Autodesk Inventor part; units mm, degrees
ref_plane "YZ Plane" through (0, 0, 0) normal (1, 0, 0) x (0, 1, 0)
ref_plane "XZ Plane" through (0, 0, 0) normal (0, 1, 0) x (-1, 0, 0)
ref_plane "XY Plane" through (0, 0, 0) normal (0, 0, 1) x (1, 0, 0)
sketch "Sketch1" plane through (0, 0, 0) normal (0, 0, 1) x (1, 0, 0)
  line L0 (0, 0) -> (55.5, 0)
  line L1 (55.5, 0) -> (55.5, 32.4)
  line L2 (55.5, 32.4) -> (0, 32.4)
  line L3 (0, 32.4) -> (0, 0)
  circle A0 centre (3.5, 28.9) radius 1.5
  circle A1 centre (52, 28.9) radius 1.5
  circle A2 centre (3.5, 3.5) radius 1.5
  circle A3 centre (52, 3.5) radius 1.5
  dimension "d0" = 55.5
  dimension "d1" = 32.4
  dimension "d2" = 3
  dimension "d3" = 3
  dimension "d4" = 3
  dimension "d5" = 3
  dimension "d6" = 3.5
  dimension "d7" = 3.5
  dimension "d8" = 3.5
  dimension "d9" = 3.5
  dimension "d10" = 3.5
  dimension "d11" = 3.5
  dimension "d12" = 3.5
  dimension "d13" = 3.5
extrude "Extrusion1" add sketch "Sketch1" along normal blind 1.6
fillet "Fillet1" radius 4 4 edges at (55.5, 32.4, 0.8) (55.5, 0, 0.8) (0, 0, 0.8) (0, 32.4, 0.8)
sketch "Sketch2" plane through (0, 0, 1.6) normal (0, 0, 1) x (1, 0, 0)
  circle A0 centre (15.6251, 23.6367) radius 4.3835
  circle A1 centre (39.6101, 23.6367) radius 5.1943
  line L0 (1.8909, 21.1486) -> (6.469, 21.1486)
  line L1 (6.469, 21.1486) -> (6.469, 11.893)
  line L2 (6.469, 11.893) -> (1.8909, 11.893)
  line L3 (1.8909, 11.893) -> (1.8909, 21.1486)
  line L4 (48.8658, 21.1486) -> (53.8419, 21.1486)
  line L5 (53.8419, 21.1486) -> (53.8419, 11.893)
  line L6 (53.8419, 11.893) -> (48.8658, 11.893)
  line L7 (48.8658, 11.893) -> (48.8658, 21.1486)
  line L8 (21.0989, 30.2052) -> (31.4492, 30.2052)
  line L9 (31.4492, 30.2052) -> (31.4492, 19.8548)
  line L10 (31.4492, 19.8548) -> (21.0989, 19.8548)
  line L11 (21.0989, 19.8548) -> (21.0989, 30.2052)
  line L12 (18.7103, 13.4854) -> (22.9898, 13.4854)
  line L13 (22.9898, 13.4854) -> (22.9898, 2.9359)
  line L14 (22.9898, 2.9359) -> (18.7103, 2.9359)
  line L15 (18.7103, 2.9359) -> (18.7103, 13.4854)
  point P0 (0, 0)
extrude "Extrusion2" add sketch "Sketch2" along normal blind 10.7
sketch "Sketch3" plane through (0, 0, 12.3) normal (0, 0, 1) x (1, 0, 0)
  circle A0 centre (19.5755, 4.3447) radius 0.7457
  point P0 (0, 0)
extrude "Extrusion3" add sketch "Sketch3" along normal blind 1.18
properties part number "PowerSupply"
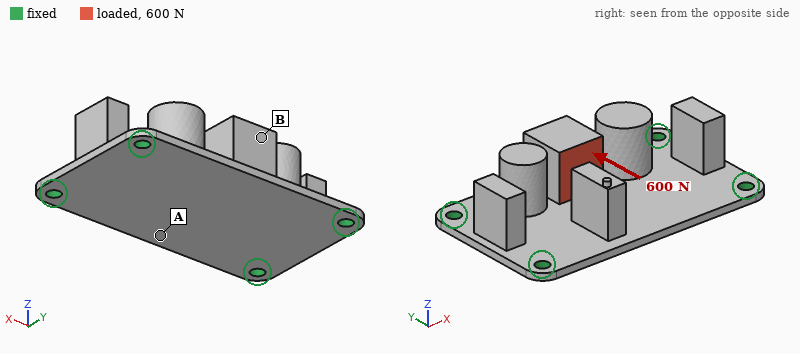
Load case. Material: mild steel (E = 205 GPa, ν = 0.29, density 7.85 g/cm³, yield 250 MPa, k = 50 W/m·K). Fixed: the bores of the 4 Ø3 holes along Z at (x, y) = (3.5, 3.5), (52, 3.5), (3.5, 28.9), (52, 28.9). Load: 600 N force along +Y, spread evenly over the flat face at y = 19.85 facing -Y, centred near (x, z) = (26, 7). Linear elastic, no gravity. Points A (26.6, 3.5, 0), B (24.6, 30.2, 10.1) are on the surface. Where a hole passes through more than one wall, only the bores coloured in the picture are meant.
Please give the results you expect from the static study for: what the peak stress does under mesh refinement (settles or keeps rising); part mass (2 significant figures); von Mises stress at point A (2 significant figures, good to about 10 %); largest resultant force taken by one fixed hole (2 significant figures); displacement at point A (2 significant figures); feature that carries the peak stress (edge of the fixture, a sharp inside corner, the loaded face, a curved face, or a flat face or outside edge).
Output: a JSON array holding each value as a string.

["keeps rising", "54 g", "36 MPa", "240 N", "29 µm", "edge of the fixture"]
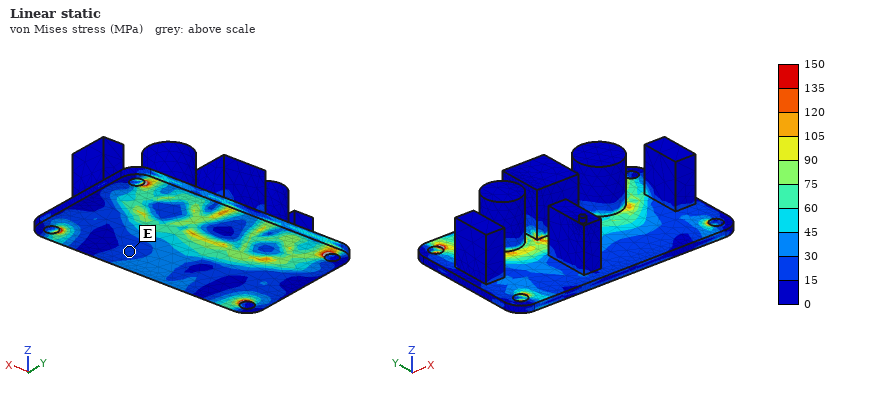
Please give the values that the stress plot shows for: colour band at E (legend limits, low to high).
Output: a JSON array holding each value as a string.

["15 to 30 MPa"]
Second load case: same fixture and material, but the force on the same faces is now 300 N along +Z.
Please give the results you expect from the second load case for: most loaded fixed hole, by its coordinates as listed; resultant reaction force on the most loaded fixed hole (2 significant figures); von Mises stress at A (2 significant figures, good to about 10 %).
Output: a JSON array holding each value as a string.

["(3.5, 28.9)", "130 N", "53 MPa"]
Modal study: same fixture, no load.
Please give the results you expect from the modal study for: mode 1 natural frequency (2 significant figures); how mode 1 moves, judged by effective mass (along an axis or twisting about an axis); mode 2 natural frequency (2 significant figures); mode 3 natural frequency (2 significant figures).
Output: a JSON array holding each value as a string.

["2200 Hz", "along Z", "3500 Hz", "5200 Hz"]
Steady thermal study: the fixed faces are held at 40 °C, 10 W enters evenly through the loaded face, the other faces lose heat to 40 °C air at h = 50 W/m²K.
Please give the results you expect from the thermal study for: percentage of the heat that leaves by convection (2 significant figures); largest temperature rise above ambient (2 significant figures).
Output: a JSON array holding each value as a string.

["45 %", "52 K"]
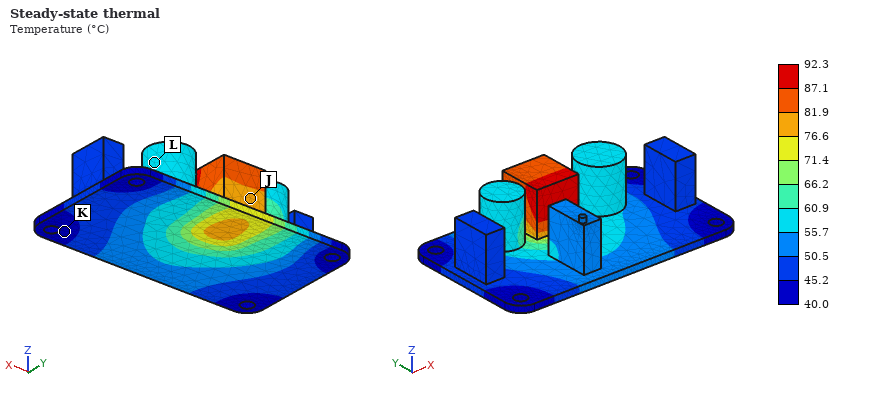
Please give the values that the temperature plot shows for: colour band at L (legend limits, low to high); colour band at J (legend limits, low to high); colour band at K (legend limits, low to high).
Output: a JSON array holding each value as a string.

["55.7 to 60.9 °C", "76.6 to 81.9 °C", "40.0 to 45.2 °C"]
